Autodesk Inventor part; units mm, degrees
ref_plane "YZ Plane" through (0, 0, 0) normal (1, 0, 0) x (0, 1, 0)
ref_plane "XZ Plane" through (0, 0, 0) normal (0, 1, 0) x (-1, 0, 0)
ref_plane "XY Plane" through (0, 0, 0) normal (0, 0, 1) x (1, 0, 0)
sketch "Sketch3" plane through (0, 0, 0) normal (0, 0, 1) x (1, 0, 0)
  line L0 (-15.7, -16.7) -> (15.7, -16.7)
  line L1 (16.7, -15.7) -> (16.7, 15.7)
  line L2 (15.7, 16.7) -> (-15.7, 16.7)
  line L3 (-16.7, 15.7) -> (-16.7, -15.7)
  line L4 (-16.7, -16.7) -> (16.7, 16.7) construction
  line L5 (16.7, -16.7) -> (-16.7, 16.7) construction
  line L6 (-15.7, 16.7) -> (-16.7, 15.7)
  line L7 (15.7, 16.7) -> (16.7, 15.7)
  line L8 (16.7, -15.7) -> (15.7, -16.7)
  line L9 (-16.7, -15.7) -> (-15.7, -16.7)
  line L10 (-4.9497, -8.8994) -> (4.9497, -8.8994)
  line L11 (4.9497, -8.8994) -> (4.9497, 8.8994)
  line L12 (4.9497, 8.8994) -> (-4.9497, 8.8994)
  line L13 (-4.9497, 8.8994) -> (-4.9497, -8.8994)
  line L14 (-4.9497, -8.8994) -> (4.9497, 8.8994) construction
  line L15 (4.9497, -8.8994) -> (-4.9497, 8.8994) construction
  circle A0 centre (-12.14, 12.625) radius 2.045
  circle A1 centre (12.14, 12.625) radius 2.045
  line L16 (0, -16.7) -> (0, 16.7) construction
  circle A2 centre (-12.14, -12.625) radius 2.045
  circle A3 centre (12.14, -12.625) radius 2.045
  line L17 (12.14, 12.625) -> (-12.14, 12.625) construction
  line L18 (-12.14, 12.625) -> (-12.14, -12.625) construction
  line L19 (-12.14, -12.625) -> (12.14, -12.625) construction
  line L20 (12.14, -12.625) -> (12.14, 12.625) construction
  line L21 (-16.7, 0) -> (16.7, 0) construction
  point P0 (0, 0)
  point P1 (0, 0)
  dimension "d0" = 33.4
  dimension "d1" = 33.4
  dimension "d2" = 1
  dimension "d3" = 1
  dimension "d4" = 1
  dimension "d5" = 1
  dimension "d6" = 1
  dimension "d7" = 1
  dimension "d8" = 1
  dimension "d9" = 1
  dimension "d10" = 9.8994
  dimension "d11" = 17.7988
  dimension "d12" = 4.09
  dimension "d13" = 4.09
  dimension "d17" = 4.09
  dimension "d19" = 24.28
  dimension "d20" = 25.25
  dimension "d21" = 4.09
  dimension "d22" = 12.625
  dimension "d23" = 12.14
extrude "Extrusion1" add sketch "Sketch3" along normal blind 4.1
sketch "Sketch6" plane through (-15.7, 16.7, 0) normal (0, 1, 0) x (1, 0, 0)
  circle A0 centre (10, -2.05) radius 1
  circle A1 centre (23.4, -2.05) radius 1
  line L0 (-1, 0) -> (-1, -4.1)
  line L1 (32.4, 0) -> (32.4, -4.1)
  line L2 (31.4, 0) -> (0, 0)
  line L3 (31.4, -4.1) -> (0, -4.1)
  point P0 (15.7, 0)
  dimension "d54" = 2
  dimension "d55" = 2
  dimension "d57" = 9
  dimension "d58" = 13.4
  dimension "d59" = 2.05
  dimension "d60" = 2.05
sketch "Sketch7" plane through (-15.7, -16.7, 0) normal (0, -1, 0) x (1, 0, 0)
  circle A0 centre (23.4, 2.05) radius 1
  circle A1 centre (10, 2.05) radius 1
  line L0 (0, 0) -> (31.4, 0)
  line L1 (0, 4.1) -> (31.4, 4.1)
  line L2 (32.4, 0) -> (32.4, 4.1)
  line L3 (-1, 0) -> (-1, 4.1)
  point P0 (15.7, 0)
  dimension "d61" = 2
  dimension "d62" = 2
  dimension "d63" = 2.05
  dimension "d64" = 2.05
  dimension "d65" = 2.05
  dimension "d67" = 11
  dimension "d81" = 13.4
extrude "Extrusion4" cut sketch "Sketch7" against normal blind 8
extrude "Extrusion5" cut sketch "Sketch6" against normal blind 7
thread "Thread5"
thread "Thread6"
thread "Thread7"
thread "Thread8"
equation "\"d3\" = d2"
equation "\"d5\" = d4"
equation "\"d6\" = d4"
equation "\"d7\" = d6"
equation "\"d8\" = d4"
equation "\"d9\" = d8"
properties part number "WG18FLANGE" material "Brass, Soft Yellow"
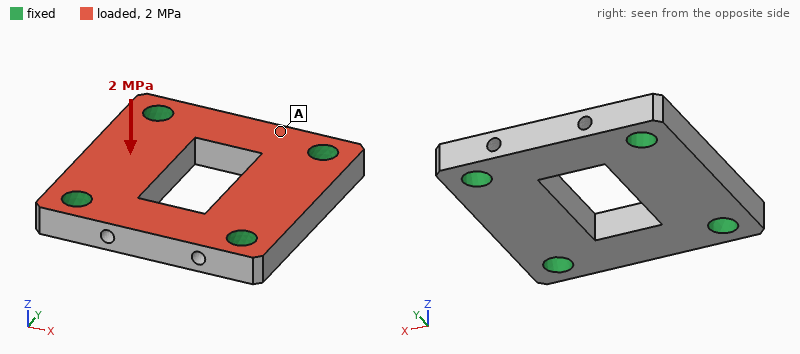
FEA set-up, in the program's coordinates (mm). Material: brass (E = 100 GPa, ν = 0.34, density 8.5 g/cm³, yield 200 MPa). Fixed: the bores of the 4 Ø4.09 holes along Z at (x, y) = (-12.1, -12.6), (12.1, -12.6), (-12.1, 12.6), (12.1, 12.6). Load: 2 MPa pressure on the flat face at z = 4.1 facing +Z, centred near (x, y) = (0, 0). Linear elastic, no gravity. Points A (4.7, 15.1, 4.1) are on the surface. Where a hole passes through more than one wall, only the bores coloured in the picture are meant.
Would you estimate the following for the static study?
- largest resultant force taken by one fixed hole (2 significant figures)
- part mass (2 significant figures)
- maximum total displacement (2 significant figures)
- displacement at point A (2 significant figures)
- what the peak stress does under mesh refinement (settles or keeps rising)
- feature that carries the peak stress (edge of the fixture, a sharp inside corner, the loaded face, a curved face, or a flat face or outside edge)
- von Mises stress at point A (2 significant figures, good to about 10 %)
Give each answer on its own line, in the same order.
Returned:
450 N
30 g
6.3 µm
2.6 µm
keeps rising
edge of the fixture
6.9 MPa
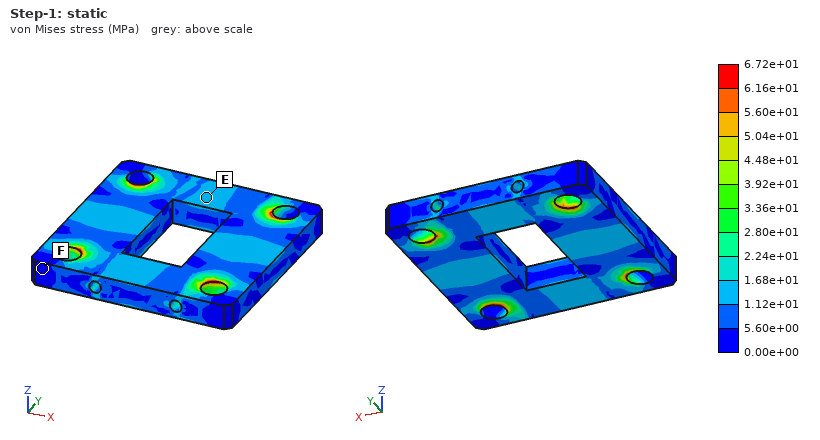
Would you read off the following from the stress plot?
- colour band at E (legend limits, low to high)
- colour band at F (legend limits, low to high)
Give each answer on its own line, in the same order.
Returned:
1.12e+01 to 1.68e+01 MPa
0.00e+00 to 5.60e+00 MPa
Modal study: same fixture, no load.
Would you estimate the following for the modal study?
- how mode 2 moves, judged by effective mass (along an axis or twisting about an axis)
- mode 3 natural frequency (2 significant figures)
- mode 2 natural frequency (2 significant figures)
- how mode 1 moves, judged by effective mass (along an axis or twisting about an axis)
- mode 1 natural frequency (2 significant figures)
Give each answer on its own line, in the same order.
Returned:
twisting about Y
24 kHz
22 kHz
along Z
20 kHz
